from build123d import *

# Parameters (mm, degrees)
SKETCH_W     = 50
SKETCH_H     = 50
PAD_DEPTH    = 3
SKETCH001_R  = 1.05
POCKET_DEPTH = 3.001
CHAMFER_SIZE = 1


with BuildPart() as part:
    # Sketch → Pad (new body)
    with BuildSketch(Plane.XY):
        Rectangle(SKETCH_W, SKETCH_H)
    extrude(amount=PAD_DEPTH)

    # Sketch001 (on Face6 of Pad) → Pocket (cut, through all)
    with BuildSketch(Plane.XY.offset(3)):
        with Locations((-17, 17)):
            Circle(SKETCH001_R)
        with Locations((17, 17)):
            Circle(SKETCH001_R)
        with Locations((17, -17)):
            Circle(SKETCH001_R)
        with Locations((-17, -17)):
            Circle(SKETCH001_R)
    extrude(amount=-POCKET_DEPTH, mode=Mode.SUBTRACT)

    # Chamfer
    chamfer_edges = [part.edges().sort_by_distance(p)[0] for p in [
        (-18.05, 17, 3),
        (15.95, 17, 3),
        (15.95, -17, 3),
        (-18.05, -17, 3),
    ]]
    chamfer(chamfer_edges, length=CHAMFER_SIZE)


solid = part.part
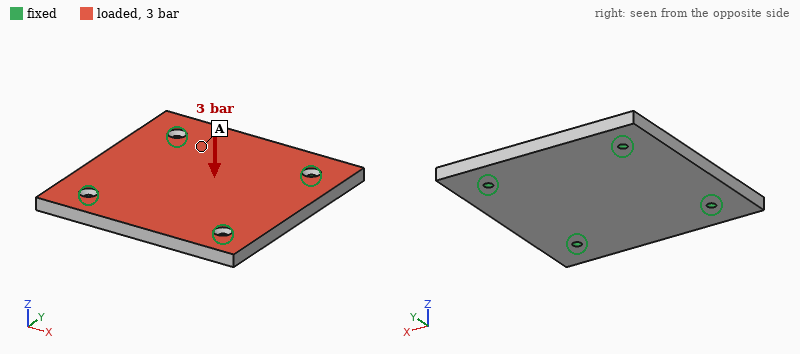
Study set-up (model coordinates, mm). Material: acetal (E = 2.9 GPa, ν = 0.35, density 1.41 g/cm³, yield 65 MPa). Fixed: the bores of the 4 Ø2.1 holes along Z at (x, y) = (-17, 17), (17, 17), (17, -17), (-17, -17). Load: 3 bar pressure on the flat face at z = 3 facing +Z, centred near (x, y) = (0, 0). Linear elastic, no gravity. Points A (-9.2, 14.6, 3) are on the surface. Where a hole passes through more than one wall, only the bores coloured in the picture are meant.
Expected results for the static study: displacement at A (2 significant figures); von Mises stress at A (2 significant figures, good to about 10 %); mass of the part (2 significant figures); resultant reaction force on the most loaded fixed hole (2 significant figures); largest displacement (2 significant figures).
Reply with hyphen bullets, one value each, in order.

- 0.23 mm
- 8.8 MPa
- 10 g
- 200 N
- 0.50 mm
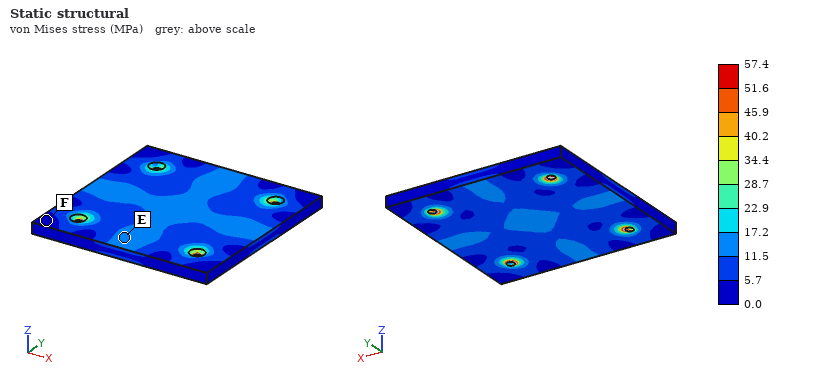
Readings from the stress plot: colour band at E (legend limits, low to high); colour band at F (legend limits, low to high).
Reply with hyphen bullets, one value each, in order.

- 11.5 to 17.2 MPa
- 0.0 to 5.7 MPa
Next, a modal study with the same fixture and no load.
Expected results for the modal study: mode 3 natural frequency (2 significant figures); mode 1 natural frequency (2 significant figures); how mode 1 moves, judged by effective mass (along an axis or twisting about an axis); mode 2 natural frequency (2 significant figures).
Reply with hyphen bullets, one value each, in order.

- 3100 Hz
- 2200 Hz
- along Z
- 2800 Hz
